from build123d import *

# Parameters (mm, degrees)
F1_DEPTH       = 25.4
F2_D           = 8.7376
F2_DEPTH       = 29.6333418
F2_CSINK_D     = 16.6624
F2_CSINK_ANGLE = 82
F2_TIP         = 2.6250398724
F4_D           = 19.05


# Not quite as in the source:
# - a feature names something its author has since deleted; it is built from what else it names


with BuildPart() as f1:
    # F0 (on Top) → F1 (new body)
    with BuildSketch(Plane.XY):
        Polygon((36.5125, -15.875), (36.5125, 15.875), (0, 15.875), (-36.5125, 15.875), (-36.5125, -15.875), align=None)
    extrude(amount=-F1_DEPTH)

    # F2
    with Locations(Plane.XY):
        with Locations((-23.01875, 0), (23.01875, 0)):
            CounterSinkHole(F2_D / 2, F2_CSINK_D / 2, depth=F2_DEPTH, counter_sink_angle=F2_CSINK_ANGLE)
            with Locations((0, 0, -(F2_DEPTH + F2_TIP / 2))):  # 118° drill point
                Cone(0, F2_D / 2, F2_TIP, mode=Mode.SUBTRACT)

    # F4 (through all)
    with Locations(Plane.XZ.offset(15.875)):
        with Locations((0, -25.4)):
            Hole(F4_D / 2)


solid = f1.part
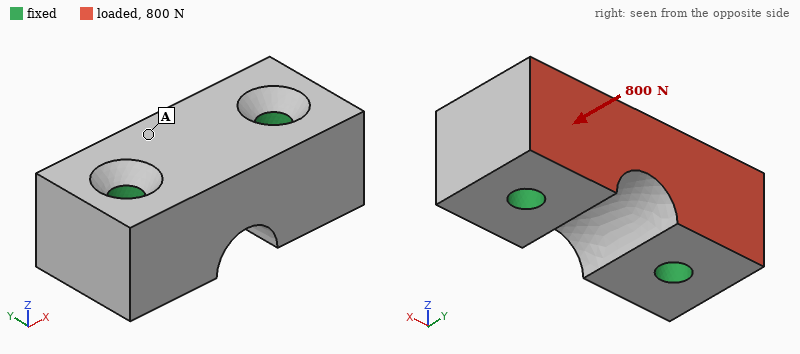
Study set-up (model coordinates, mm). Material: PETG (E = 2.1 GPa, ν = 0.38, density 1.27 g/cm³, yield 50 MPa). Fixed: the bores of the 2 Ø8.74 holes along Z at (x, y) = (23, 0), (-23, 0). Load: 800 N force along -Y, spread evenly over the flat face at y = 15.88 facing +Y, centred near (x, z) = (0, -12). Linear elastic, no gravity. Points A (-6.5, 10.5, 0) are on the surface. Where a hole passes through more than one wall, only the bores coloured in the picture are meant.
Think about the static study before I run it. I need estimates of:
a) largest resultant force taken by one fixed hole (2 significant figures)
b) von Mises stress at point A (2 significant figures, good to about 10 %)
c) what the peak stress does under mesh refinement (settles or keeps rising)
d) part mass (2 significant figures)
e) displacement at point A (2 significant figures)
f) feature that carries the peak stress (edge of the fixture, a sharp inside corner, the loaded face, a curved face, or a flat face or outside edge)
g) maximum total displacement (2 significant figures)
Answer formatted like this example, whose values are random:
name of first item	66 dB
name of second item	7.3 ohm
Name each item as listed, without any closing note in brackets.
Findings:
largest resultant force taken by one fixed hole	400 N
von Mises stress at point A	0.41 MPa
what the peak stress does under mesh refinement	keeps rising
part mass	64 g
displacement at point A	10 µm
feature that carries the peak stress	edge of the fixture
maximum total displacement	12 µm
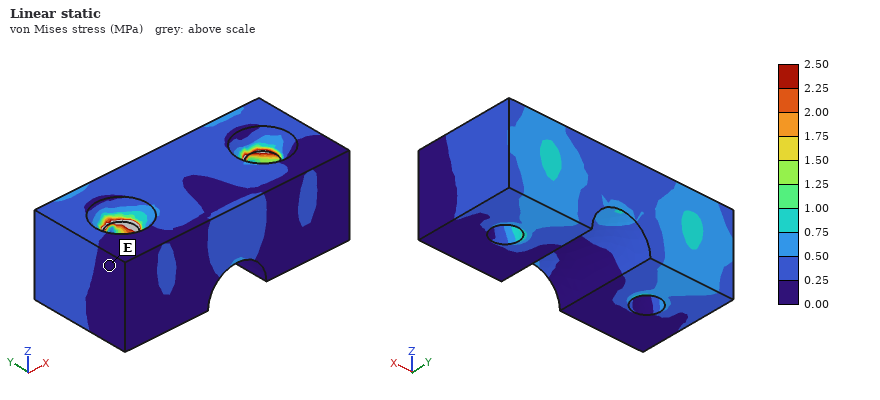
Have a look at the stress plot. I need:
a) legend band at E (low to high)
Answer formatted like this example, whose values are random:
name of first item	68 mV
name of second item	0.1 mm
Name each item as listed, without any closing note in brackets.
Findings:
legend band at E	0.00 to 0.25 MPa
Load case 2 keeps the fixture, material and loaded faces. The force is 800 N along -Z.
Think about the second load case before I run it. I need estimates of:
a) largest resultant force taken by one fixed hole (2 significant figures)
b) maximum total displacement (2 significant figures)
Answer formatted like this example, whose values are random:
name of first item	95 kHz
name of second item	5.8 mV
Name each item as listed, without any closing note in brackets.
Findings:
largest resultant force taken by one fixed hole	400 N
maximum total displacement	38 µm
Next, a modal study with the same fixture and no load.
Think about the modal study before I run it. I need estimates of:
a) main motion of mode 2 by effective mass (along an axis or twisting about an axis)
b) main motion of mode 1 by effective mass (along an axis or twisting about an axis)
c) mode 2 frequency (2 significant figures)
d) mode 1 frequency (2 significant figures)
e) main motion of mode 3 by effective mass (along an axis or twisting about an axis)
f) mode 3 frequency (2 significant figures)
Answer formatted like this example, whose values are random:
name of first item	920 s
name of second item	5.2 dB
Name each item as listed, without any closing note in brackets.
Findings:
main motion of mode 2 by effective mass	along Z
main motion of mode 1 by effective mass	along Y
mode 2 frequency	6800 Hz
mode 1 frequency	5900 Hz
main motion of mode 3 by effective mass	twisting about X
mode 3 frequency	7200 Hz
